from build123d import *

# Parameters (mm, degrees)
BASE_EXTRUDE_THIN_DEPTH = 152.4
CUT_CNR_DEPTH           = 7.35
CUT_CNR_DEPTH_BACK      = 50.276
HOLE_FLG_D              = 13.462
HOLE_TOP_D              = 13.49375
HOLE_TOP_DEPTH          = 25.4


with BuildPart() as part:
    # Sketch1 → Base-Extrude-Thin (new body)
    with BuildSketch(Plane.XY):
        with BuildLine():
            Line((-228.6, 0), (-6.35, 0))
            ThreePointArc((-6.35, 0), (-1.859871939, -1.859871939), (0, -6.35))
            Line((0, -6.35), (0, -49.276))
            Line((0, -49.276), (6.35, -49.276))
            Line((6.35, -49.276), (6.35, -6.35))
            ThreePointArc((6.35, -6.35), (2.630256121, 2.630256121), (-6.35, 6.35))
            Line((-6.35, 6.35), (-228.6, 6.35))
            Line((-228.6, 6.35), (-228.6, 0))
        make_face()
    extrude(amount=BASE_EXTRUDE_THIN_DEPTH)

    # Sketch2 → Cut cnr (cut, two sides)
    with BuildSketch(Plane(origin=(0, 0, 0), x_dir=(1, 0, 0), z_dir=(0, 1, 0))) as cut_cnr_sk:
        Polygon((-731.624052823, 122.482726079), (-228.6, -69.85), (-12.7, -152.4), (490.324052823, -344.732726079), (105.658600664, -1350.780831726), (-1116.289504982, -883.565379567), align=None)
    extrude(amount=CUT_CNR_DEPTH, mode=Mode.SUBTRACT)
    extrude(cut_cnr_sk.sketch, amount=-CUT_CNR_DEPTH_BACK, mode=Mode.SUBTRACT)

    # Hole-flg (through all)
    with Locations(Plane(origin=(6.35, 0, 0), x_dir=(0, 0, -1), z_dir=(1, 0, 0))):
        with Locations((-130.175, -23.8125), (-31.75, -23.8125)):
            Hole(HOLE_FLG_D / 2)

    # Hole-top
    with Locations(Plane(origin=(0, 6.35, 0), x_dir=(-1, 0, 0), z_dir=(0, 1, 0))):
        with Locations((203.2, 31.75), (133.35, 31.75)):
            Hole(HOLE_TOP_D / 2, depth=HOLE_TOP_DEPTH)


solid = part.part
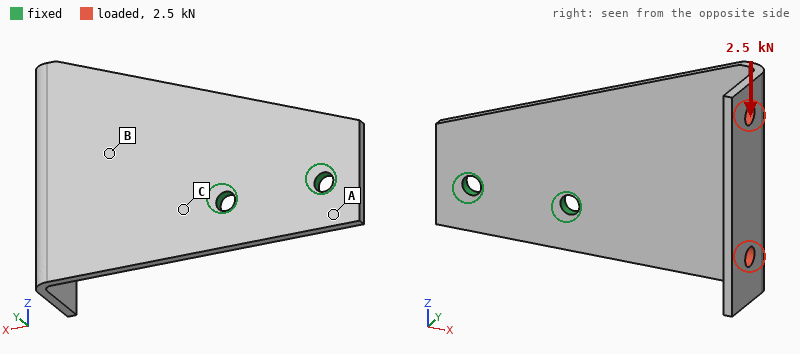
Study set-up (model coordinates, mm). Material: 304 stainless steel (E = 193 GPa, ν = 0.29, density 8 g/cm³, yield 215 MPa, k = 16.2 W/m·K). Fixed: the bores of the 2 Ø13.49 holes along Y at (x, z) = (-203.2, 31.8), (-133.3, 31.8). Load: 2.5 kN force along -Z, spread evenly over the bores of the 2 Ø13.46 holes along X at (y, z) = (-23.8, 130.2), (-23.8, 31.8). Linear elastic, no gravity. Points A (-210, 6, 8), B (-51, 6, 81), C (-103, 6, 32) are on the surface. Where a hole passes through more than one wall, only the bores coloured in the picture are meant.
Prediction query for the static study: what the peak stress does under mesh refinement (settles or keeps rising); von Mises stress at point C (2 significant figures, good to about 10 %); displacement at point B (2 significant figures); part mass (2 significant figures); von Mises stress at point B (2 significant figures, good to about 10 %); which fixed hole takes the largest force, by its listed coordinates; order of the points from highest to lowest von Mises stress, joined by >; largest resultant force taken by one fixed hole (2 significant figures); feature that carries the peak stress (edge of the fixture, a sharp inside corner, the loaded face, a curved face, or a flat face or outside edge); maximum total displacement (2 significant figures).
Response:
keeps rising
78 MPa
0.34 mm
1.7 kg
46 MPa
(-133.3, 31.8)
C > B > A
6.7 kN
edge of the fixture
1.5 mm
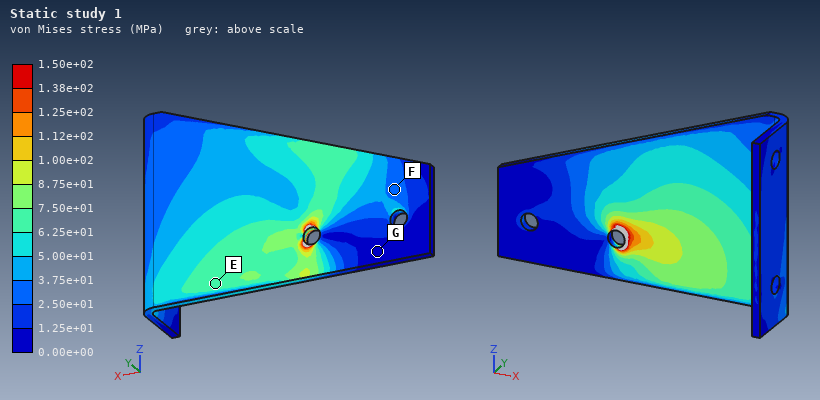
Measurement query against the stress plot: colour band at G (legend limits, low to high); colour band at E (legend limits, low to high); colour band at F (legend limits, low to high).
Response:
0.00e+00 to 1.25e+01 MPa
6.25e+01 to 7.50e+01 MPa
2.50e+01 to 3.75e+01 MPa
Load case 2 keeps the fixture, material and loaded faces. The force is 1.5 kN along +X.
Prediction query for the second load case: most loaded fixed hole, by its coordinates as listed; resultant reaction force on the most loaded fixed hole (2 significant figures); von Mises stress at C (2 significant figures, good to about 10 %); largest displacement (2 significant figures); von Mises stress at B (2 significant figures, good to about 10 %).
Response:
(-133.3, 31.8)
1.3 kN
51 MPa
1.1 mm
39 MPa
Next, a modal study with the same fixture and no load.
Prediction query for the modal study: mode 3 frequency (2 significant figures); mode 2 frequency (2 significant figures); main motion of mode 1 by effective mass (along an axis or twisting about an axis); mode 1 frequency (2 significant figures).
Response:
710 Hz
300 Hz
along Y
130 Hz
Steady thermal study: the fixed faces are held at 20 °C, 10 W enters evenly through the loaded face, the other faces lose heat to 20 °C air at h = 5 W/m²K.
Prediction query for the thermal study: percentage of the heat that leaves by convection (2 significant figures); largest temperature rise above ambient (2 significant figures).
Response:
79 %
63 K
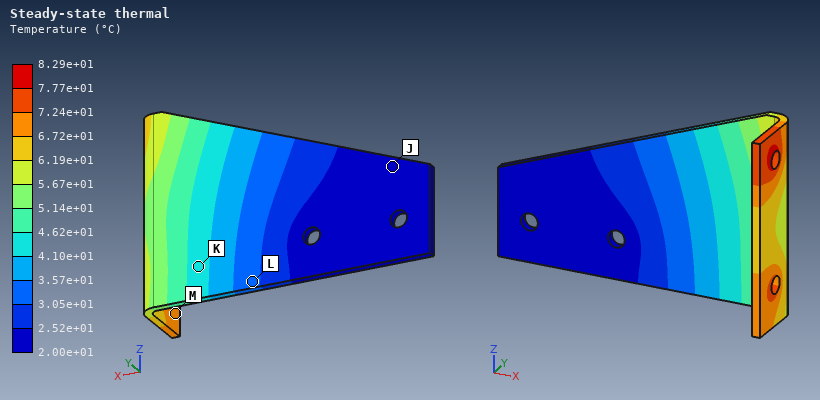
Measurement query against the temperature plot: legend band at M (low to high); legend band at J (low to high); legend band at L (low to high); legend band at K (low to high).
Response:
6.72e+01 to 7.24e+01 °C
2.00e+01 to 2.52e+01 °C
3.05e+01 to 3.57e+01 °C
4.10e+01 to 4.62e+01 °C
